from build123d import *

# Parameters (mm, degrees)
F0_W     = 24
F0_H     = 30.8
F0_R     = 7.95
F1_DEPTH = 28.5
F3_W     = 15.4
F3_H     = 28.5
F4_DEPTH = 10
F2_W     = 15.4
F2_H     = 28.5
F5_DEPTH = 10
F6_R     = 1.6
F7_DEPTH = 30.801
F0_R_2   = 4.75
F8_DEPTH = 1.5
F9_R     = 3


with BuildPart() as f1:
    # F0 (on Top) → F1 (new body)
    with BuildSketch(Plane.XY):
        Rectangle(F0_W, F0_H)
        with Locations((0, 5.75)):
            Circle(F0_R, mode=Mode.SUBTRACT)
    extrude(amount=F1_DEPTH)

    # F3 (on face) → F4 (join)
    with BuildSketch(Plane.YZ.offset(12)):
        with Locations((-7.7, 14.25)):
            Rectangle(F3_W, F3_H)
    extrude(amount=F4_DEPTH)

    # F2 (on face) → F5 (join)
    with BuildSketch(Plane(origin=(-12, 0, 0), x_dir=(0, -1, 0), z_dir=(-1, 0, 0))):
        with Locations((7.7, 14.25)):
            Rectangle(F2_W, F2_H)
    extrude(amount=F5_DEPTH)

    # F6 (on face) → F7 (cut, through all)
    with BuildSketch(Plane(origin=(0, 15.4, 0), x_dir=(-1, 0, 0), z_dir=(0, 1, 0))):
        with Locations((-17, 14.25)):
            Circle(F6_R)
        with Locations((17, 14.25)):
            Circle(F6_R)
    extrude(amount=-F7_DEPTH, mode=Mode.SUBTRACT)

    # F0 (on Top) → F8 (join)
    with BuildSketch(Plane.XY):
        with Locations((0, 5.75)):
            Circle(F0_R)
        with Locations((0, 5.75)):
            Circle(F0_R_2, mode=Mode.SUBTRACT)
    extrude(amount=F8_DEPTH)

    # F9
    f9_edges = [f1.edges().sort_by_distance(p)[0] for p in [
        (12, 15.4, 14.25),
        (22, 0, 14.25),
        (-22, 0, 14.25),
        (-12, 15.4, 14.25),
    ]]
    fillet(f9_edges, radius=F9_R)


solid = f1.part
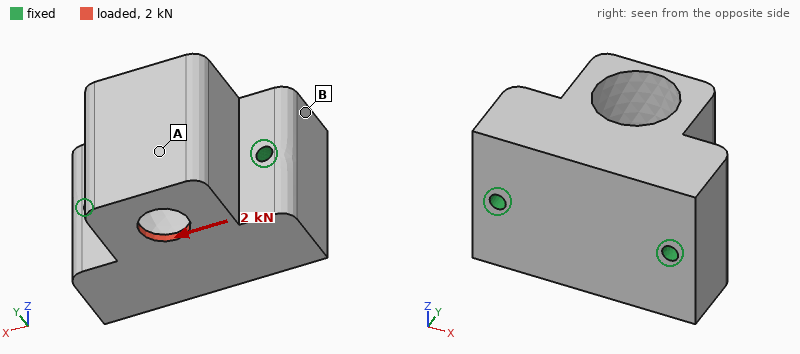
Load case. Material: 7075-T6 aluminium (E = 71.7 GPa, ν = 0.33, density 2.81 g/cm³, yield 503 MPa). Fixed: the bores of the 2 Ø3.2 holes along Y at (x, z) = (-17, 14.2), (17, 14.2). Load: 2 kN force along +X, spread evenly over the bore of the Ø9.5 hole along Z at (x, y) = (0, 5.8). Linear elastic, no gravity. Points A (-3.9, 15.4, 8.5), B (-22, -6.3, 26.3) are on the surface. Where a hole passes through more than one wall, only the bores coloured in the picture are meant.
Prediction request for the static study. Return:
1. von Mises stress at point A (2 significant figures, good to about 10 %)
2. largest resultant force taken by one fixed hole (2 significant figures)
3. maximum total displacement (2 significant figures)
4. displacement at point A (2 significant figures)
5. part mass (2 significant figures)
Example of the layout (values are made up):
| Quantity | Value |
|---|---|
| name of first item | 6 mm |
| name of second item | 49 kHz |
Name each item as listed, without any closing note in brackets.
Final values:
| Quantity | Value |
|---|---|
| von Mises stress at point A | 19 MPa |
| largest resultant force taken by one fixed hole | 1.5 kN |
| maximum total displacement | 21 µm |
| displacement at point A | 12 µm |
| part mass | 67 g |
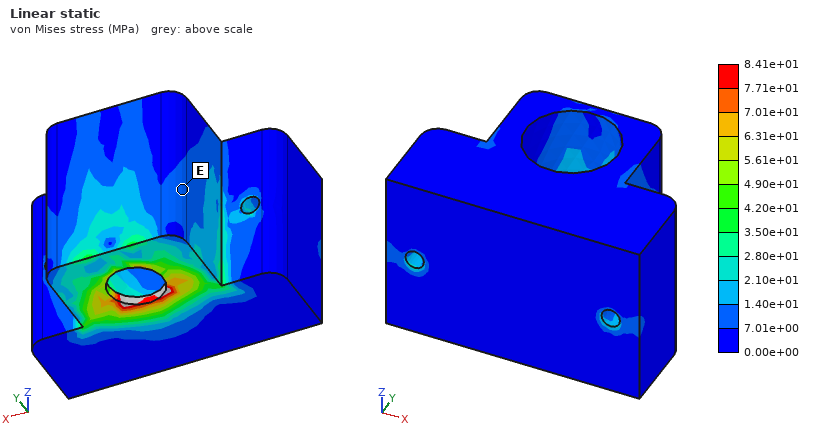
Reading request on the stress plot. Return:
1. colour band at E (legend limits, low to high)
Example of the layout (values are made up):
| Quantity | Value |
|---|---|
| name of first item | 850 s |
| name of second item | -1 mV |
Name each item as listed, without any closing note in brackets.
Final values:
| Quantity | Value |
|---|---|
| colour band at E | 7.01e+00 to 1.40e+01 MPa |
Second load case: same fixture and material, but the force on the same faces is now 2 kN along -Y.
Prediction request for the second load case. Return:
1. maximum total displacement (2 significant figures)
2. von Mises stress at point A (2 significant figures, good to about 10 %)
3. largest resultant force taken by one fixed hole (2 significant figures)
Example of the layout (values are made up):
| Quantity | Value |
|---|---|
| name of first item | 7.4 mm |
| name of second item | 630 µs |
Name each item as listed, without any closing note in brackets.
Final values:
| Quantity | Value |
|---|---|
| maximum total displacement | 21 µm |
| von Mises stress at point A | 11 MPa |
| largest resultant force taken by one fixed hole | 1.0 kN |
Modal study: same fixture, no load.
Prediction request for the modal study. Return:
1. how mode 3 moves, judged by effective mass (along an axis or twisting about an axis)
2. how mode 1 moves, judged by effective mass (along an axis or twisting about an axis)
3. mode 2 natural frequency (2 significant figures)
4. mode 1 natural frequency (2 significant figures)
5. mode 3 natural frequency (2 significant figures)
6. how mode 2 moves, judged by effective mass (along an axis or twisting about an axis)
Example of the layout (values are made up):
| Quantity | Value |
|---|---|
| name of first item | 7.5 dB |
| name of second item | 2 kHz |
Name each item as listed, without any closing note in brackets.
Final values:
| Quantity | Value |
|---|---|
| how mode 3 moves, judged by effective mass | along Y |
| how mode 1 moves, judged by effective mass | along Z |
| mode 2 natural frequency | 16 kHz |
| mode 1 natural frequency | 14 kHz |
| mode 3 natural frequency | 23 kHz |
| how mode 2 moves, judged by effective mass | along X |
